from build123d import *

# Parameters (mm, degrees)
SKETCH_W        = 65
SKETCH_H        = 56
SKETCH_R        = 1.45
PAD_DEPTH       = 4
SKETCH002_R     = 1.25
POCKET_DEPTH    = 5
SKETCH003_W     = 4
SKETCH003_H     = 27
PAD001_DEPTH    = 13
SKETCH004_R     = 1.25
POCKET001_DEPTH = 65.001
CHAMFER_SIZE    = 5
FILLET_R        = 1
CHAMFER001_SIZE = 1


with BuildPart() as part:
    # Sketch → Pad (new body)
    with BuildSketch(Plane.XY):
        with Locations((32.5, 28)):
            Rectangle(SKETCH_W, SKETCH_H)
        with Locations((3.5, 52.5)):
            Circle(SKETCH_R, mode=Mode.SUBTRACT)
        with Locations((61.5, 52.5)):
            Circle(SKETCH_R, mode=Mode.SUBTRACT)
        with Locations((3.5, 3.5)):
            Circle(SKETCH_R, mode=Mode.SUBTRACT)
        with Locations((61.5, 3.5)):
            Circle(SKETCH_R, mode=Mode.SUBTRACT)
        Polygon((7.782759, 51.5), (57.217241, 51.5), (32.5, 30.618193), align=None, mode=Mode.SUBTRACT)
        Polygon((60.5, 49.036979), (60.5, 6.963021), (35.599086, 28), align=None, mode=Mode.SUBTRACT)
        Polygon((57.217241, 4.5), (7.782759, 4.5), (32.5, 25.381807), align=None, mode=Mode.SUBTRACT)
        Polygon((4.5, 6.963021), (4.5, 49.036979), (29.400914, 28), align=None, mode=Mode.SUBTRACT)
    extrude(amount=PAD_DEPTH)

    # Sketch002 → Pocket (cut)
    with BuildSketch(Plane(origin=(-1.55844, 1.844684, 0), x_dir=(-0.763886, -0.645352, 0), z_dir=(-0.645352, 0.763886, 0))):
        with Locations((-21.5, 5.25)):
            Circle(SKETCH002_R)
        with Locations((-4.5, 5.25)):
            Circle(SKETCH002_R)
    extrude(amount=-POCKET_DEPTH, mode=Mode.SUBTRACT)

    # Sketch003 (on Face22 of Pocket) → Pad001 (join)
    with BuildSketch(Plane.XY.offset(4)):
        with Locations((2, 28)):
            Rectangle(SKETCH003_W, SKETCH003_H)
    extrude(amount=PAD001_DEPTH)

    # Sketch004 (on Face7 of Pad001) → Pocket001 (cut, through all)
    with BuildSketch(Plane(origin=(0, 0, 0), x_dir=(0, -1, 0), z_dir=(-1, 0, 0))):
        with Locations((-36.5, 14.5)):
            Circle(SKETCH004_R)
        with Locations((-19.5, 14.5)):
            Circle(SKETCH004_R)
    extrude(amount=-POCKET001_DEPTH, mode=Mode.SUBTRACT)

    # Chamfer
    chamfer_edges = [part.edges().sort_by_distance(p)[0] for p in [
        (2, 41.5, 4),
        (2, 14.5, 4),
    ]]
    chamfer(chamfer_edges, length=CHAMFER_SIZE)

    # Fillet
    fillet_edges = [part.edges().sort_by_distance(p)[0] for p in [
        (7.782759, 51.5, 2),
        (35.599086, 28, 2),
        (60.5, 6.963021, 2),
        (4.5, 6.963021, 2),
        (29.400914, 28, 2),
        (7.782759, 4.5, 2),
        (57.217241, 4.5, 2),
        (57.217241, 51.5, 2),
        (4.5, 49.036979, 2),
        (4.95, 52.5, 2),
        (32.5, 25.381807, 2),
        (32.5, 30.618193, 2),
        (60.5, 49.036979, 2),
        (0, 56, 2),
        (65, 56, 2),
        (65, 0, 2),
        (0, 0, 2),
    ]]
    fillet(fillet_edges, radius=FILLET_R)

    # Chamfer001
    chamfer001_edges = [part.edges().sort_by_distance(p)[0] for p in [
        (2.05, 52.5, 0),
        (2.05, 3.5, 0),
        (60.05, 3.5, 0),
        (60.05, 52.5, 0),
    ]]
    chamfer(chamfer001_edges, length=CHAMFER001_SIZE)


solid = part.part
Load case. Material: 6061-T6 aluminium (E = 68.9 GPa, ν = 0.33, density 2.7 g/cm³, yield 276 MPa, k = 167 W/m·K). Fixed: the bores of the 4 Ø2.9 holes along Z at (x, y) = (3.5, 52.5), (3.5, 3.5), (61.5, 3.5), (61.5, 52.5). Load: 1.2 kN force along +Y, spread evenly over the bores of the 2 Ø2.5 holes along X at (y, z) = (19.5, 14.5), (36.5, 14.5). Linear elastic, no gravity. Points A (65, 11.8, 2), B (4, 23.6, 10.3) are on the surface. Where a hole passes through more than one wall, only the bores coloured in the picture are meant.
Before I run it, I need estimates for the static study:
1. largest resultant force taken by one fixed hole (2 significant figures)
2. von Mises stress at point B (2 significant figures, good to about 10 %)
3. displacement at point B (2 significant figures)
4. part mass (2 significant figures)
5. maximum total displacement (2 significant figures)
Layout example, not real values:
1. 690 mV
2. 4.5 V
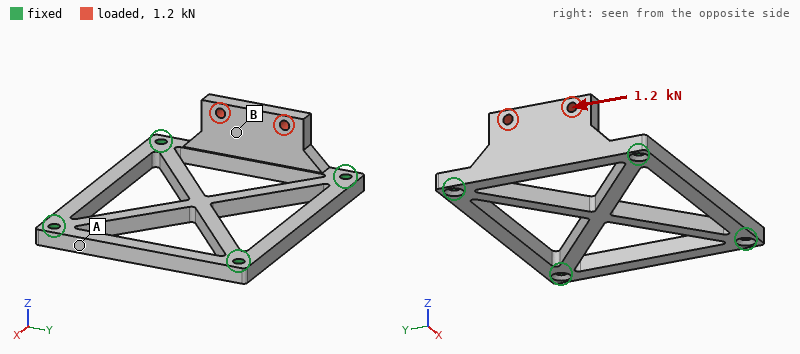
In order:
1. 700 N
2. 20 MPa
3. 15 µm
4. 21 g
5. 29 µm
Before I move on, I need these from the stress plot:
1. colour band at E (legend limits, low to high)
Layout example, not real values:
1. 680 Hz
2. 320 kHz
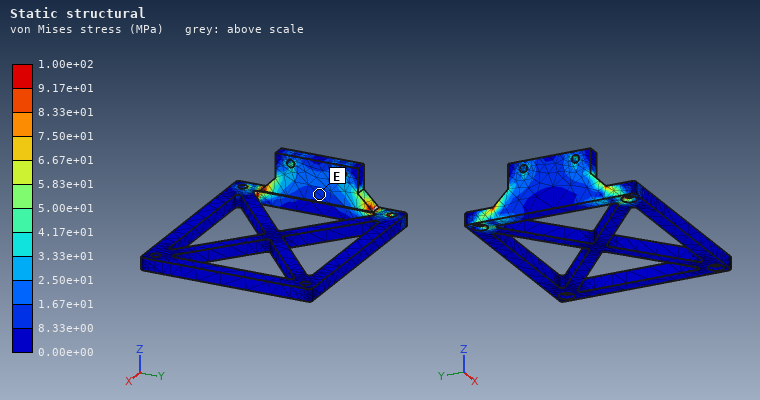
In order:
1. 8.33e+00 to 1.67e+01 MPa
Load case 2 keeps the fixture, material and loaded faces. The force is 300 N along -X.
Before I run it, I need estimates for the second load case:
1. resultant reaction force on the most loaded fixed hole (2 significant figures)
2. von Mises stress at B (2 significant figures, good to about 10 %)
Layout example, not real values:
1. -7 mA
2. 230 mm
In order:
1. 180 N
2. 28 MPa
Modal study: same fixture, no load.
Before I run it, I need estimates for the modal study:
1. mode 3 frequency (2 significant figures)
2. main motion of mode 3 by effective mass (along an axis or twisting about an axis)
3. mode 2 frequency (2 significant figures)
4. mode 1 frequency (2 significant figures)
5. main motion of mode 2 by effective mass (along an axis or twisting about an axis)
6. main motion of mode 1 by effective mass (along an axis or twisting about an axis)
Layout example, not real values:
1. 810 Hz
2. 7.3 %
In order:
1. 6500 Hz
2. twisting about X
3. 4500 Hz
4. 4000 Hz
5. along X
6. along Z
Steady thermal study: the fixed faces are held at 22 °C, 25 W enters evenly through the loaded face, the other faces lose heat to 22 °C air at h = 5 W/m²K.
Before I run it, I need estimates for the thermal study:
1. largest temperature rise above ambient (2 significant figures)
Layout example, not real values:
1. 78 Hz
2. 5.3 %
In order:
1. 59 K
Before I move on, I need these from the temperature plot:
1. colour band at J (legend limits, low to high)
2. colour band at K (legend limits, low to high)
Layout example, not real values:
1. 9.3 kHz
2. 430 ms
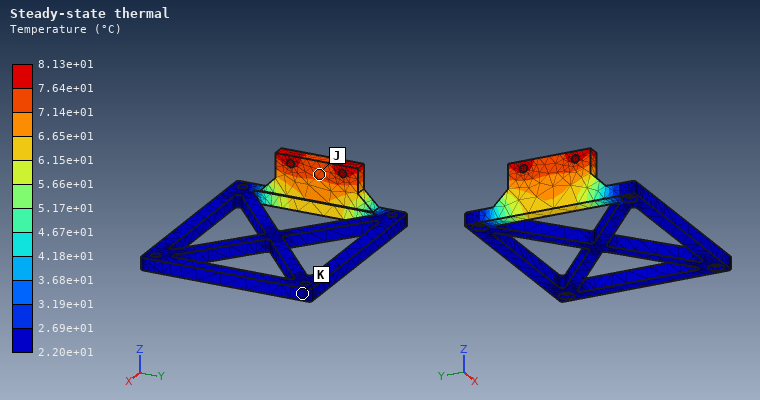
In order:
1. 7.14e+01 to 7.64e+01 °C
2. 2.20e+01 to 2.69e+01 °C
